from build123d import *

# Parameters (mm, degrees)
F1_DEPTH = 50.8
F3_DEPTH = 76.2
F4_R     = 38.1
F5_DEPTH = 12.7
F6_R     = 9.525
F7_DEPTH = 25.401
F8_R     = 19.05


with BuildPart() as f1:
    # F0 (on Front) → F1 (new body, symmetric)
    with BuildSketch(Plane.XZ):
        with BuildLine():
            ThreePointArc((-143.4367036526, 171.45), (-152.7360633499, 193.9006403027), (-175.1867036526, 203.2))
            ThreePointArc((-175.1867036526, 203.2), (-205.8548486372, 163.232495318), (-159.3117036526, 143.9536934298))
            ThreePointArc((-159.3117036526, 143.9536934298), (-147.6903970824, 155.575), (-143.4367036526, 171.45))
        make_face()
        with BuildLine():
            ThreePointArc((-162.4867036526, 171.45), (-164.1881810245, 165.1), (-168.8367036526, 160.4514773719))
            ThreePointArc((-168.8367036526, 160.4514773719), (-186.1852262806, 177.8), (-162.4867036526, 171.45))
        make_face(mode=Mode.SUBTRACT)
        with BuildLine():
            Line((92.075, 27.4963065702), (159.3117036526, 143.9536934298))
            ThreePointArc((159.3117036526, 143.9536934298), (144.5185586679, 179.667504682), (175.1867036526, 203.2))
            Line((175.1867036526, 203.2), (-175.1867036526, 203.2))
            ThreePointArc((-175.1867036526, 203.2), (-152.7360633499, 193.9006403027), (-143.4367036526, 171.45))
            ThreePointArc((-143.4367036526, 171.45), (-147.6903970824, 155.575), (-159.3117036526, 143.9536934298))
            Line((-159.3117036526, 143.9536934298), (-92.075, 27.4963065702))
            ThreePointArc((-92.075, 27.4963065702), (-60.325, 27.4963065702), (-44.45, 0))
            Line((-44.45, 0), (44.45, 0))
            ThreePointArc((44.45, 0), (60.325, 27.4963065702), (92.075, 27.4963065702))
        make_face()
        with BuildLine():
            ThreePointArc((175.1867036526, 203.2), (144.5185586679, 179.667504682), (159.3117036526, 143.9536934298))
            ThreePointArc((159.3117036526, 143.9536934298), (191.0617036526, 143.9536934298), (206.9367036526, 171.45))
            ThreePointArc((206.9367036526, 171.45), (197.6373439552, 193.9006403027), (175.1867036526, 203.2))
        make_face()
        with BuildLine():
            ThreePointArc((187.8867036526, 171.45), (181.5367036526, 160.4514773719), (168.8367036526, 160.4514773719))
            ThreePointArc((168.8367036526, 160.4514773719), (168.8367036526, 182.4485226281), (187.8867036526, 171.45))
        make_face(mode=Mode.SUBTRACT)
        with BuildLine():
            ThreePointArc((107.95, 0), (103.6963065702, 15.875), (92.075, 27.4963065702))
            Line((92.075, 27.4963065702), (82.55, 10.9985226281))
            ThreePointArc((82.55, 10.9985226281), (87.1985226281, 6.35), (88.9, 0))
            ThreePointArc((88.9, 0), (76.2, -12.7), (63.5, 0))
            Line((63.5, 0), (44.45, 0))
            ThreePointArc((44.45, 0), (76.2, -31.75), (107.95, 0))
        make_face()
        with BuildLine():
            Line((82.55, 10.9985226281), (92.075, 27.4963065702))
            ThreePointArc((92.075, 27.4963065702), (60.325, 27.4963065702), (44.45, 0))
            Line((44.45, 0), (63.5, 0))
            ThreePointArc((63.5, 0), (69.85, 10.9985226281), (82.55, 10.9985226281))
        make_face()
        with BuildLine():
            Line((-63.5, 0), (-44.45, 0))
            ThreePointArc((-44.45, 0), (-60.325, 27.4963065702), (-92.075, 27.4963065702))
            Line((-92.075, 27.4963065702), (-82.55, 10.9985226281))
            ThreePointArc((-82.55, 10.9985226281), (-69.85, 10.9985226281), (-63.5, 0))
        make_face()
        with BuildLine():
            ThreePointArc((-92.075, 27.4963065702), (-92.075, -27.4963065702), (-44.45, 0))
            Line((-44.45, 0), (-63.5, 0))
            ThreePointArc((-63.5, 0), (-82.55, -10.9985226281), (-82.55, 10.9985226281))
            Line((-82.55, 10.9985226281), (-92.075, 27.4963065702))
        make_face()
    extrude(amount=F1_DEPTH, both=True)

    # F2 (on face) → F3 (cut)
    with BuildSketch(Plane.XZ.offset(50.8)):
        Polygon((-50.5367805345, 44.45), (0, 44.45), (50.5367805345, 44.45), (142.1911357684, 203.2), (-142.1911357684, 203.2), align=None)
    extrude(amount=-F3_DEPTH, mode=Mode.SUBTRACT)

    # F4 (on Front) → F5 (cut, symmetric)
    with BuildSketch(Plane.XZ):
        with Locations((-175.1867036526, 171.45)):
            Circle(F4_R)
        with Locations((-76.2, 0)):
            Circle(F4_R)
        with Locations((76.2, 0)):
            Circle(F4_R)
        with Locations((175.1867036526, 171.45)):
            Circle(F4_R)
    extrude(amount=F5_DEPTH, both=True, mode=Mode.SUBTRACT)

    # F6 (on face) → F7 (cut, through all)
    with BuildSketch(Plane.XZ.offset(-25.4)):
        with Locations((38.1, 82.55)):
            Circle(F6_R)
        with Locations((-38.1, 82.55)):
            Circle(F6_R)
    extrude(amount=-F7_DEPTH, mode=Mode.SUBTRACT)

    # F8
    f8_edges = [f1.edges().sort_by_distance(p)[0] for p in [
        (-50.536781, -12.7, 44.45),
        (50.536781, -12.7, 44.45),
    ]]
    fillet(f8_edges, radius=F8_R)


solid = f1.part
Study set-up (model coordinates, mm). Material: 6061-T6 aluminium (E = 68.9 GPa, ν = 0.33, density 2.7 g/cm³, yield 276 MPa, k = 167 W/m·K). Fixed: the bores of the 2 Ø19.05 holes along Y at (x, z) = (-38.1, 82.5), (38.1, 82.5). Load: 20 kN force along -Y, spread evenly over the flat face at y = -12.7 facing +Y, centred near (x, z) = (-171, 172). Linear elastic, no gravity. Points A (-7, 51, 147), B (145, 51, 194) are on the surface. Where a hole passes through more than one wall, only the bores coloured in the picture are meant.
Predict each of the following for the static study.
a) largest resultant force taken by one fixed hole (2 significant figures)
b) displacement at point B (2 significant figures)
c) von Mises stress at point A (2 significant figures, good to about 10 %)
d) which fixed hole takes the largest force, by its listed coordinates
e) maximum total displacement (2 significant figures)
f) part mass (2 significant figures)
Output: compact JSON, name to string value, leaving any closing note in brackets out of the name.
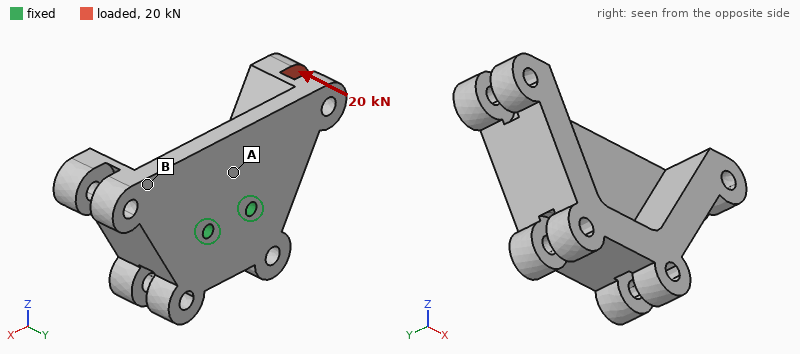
{"largest resultant force taken by one fixed hole": "41 kN", "displacement at point B": "0.14 mm", "von Mises stress at point A": "23 MPa", "which fixed hole takes the largest force, by its listed coordinates": "(-38.1, 82.5)", "maximum total displacement": "0.84 mm", "part mass": "9.3 kg"}
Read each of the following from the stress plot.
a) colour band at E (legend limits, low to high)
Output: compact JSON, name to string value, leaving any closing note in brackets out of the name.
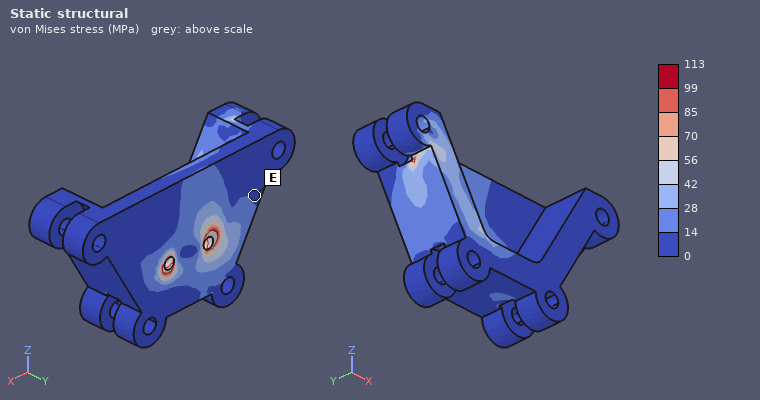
{"colour band at E": "0 to 14 MPa"}
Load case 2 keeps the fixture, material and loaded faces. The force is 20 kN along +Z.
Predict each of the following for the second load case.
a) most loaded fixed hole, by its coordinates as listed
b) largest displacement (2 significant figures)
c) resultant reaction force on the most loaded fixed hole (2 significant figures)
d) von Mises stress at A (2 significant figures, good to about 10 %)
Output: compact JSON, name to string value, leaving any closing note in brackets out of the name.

{"most loaded fixed hole, by its coordinates as listed": "(-38.1, 82.5)", "largest displacement": "0.46 mm", "resultant reaction force on the most loaded fixed hole": "48 kN", "von Mises stress at A": "18 MPa"}
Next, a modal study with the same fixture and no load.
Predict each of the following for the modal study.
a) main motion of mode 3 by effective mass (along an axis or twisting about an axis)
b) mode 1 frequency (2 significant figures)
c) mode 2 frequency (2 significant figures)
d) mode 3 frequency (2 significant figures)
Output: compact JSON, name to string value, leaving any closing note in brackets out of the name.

{"main motion of mode 3 by effective mass": "twisting about Y", "mode 1 frequency": "630 Hz", "mode 2 frequency": "820 Hz", "mode 3 frequency": "1100 Hz"}
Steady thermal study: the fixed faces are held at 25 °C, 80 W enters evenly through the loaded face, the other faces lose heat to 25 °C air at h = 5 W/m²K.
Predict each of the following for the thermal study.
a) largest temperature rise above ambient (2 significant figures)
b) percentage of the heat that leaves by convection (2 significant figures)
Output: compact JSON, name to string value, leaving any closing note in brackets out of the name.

{"largest temperature rise above ambient": "27 K", "percentage of the heat that leaves by convection": "8.4 %"}
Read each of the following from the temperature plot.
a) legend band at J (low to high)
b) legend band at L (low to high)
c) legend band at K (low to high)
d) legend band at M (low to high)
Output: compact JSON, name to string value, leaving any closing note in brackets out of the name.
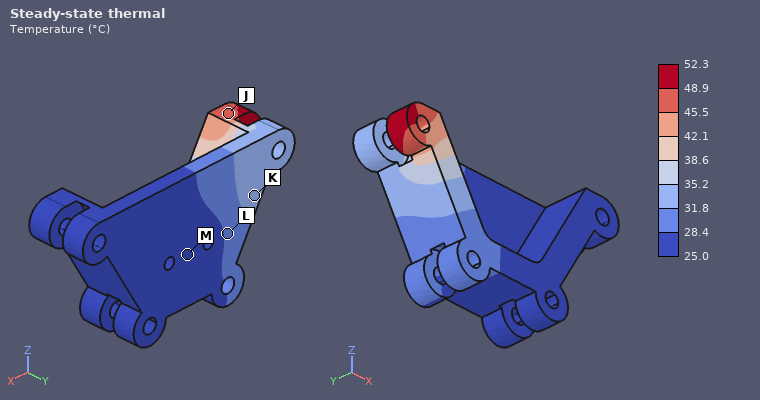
{"legend band at J": "45.5 to 48.9 °C", "legend band at L": "28.4 to 31.8 °C", "legend band at K": "31.8 to 35.2 °C", "legend band at M": "25.0 to 28.4 °C"}
